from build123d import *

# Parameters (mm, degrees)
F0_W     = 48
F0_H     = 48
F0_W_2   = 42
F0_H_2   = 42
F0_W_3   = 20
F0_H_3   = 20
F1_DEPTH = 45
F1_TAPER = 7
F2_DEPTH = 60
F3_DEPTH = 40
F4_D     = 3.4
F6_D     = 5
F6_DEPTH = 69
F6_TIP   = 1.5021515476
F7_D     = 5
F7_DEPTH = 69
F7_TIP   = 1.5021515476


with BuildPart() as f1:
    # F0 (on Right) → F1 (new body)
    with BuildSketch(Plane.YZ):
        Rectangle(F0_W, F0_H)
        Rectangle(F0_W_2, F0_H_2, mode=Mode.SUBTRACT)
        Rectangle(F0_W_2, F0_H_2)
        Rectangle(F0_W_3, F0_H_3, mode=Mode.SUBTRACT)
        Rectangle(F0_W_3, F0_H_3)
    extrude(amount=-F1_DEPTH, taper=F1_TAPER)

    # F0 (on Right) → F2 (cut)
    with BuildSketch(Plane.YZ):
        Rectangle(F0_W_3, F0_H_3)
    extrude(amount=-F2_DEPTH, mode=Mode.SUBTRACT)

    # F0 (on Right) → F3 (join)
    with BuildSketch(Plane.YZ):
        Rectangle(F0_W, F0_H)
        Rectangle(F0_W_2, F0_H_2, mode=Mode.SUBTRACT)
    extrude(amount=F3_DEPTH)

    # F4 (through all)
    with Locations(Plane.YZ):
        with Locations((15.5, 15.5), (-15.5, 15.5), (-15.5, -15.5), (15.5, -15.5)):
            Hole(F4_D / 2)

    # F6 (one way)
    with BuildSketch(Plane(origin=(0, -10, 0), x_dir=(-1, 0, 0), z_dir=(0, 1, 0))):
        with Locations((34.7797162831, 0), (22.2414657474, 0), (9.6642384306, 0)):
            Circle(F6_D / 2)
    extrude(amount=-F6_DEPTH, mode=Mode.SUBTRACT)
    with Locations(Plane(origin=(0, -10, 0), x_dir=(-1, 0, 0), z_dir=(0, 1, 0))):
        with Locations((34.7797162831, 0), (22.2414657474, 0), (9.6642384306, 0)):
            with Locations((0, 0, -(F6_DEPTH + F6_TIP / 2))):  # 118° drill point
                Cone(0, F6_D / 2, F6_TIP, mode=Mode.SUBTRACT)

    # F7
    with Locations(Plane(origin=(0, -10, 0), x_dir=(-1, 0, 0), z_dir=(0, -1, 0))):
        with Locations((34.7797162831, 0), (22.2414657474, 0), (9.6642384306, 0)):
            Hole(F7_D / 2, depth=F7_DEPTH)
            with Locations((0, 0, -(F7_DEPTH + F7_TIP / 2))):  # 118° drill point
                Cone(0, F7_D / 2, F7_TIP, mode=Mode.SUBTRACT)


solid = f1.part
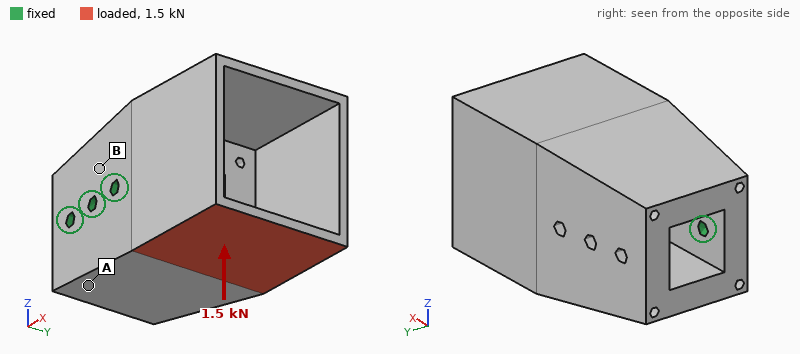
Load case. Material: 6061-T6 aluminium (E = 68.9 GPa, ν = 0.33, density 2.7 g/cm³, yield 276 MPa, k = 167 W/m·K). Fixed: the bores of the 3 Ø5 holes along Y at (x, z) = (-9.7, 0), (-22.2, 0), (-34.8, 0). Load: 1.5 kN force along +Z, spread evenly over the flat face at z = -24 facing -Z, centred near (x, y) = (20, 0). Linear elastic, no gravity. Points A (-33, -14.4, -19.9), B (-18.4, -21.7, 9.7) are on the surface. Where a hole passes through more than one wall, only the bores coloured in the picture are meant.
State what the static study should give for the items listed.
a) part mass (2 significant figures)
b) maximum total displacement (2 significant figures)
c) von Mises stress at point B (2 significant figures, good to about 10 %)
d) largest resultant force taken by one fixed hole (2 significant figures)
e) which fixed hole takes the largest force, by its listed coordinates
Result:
220 g
0.13 mm
8.5 MPa
2.9 kN
(-9.7, 0)
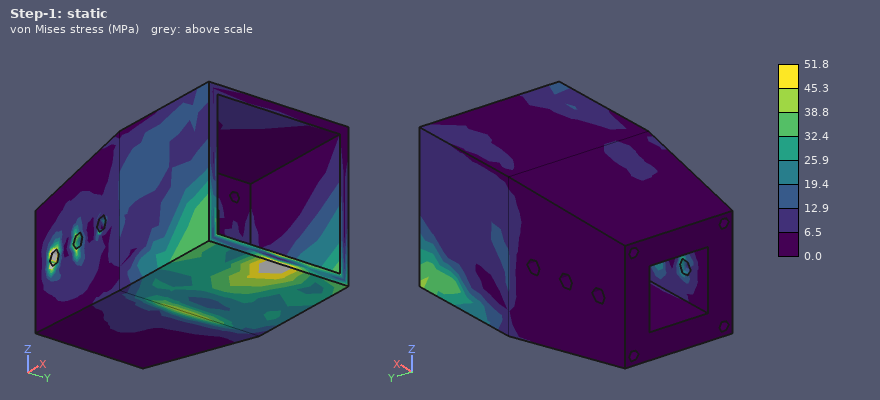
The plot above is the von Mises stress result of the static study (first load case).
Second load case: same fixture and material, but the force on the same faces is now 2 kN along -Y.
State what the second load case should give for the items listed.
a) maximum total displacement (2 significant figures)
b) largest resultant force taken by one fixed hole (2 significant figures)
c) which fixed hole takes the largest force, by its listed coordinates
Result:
85 µm
3.3 kN
(-9.7, 0)
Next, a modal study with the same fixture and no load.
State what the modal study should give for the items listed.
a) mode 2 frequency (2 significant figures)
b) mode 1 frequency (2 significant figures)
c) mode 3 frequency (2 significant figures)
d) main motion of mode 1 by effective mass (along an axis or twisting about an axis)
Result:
3800 Hz
3200 Hz
4700 Hz
along Z
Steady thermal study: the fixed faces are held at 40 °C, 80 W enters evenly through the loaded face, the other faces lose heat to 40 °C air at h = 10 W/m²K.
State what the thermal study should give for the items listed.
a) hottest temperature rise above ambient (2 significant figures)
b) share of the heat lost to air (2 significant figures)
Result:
56 K
5.5 %
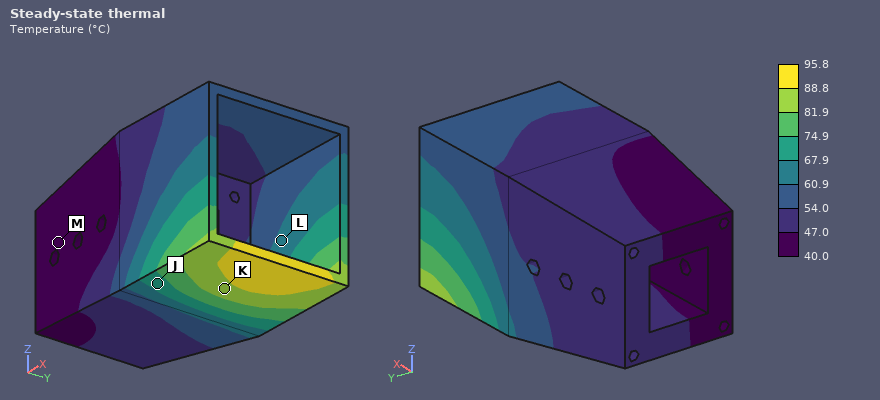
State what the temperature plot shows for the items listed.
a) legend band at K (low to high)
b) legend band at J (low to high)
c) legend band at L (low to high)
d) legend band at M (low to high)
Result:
81.9 to 88.8 °C
67.9 to 74.9 °C
60.9 to 67.9 °C
40.0 to 47.0 °C
